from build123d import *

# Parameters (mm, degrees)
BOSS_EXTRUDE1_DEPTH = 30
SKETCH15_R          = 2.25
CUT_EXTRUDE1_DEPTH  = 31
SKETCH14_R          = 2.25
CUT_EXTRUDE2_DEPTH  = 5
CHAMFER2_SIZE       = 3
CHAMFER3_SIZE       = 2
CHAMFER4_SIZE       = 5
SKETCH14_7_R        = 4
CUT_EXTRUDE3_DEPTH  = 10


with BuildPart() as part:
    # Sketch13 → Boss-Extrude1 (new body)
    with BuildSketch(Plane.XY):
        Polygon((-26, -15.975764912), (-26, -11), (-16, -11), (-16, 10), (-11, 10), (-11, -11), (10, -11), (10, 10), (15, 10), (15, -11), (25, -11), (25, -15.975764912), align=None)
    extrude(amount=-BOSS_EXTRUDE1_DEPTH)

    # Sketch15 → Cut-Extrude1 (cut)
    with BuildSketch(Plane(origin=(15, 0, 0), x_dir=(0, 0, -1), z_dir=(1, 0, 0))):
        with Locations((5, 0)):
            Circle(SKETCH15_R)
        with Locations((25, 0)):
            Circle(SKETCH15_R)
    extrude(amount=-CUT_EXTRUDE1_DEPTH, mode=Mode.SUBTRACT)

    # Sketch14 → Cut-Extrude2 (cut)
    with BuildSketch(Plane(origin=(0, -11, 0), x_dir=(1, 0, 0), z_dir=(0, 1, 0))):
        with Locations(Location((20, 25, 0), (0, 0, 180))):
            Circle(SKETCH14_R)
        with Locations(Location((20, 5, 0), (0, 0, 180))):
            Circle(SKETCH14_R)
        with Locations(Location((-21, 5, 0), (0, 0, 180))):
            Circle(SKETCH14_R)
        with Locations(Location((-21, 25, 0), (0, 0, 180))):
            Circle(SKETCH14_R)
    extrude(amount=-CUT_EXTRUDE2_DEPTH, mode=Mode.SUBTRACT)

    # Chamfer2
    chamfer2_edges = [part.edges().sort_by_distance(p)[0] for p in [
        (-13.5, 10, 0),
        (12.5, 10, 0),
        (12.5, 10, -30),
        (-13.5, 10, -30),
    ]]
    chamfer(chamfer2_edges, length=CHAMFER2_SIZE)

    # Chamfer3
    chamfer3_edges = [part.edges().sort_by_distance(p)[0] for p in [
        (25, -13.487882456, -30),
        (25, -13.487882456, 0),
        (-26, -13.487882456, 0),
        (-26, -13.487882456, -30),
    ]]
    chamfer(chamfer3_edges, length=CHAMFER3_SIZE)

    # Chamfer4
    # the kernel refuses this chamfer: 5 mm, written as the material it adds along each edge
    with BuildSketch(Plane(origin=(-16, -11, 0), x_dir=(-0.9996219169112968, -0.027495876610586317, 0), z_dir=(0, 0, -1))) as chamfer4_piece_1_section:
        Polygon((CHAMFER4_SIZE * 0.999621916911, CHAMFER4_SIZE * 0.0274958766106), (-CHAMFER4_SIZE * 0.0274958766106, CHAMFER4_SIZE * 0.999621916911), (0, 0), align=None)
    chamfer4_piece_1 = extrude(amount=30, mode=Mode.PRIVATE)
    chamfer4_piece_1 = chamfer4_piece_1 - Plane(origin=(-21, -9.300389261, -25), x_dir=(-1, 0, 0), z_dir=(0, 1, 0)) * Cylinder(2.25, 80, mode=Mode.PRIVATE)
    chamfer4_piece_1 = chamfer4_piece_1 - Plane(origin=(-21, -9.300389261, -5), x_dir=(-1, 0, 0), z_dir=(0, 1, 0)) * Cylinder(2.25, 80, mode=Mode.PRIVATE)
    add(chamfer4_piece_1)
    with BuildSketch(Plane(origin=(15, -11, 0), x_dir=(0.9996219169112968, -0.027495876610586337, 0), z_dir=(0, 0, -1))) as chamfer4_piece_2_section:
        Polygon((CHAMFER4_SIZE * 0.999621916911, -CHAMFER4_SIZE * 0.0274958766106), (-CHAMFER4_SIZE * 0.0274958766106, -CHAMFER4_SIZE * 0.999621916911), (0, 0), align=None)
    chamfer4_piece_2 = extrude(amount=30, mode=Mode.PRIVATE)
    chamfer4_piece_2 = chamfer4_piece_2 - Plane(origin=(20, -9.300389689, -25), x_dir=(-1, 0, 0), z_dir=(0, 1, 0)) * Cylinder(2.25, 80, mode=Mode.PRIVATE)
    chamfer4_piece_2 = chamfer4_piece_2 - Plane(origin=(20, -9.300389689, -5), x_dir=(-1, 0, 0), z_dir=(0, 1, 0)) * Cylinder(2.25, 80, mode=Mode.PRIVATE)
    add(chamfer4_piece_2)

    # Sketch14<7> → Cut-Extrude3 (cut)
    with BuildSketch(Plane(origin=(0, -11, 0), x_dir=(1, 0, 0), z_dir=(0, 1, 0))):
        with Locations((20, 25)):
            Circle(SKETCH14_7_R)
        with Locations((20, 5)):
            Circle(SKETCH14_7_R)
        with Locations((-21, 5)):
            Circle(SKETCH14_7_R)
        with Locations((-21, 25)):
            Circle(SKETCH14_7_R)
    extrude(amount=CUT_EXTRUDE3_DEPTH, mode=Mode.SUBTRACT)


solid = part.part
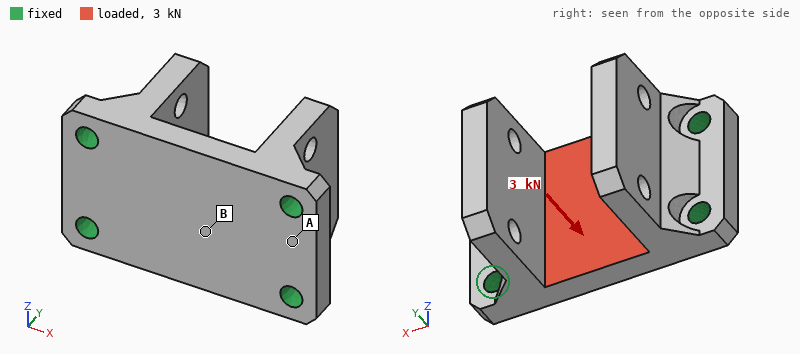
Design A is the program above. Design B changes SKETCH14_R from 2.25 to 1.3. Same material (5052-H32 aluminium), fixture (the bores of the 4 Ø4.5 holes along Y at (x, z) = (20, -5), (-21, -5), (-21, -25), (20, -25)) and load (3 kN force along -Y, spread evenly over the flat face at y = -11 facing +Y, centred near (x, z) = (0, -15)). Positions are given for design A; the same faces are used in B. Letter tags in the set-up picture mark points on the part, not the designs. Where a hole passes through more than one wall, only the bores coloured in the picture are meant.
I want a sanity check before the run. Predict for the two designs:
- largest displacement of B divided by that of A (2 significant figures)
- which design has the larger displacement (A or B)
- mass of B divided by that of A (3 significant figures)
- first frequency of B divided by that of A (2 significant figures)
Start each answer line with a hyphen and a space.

- 1.4
- B
- 1.02
- 0.90
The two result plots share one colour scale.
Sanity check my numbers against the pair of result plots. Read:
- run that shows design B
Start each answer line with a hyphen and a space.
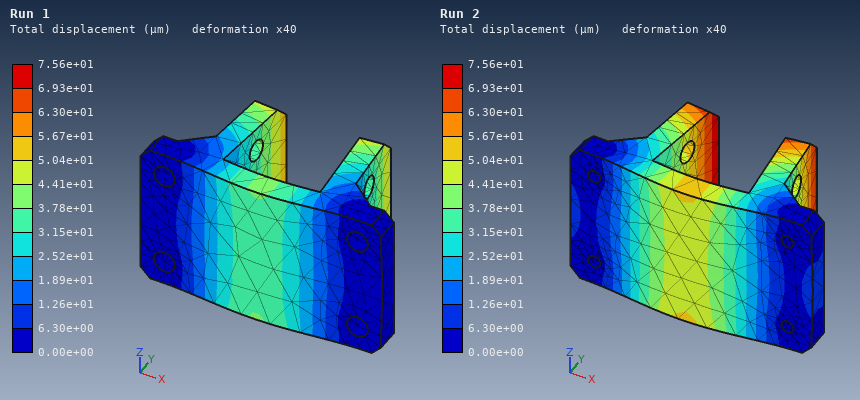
- Run 2
